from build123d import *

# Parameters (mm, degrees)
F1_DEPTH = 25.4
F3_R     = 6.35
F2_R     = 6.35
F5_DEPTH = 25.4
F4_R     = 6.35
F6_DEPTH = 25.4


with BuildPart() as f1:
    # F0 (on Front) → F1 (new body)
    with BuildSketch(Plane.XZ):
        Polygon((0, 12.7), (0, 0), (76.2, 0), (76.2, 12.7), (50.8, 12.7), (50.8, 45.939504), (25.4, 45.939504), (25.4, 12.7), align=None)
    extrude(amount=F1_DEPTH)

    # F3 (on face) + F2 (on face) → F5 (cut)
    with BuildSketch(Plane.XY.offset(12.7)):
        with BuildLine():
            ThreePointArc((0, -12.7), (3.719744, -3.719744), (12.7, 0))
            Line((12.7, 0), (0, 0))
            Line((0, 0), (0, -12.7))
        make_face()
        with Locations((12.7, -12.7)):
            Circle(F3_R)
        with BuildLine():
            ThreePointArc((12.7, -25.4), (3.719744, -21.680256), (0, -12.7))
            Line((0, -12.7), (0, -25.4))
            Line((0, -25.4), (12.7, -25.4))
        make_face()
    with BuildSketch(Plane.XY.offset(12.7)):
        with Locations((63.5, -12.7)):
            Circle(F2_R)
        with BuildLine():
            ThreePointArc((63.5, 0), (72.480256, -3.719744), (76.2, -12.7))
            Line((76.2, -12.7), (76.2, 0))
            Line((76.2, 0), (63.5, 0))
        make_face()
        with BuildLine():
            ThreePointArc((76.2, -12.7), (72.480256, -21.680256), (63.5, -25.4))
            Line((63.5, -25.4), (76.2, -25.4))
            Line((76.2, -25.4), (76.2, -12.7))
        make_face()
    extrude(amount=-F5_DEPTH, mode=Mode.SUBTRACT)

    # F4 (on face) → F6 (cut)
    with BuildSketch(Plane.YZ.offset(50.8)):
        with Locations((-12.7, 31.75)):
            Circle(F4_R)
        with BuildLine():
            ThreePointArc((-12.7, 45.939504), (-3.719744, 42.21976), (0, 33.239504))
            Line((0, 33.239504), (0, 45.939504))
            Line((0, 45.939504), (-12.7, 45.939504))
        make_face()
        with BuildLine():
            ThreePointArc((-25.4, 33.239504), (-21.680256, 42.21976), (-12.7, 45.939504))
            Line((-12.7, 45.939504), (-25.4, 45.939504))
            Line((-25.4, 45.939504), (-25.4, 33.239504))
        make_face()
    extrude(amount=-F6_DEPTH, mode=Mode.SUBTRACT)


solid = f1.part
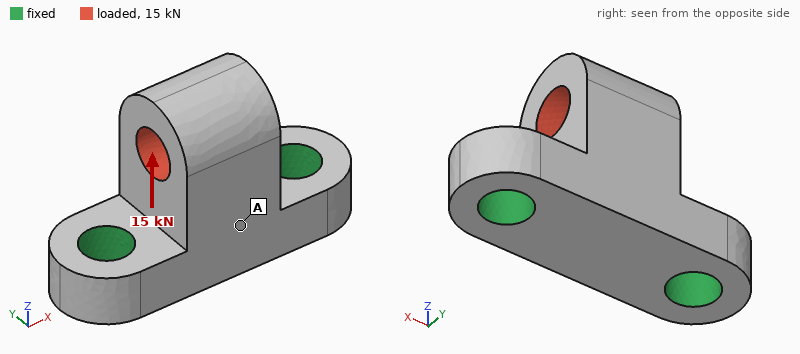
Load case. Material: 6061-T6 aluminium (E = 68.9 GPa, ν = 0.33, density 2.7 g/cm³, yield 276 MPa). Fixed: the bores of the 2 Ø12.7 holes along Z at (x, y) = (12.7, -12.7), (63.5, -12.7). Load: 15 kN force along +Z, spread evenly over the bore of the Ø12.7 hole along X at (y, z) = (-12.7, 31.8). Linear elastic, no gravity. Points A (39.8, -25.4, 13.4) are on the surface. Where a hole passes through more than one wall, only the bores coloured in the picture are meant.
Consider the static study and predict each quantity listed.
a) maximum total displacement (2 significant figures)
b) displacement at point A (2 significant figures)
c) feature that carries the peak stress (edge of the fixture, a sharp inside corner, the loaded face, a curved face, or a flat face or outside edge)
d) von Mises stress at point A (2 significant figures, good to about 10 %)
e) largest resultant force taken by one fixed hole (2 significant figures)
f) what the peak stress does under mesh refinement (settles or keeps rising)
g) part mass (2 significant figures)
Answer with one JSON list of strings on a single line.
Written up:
["33 µm", "21 µm", "edge of the fixture", "15 MPa", "7.8 kN", "keeps rising", "97 g"]
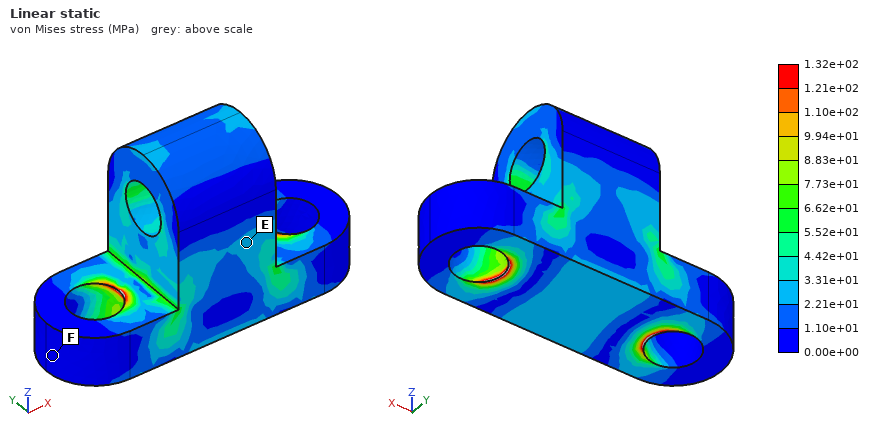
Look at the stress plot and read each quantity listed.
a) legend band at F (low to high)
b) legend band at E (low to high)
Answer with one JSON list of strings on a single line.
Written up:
["0.00e+00 to 1.10e+01 MPa", "2.21e+01 to 3.31e+01 MPa"]
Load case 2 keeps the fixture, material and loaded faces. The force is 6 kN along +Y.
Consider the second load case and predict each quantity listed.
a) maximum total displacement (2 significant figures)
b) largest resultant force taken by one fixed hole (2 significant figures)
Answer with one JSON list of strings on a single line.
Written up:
["0.14 mm", "3.0 kN"]
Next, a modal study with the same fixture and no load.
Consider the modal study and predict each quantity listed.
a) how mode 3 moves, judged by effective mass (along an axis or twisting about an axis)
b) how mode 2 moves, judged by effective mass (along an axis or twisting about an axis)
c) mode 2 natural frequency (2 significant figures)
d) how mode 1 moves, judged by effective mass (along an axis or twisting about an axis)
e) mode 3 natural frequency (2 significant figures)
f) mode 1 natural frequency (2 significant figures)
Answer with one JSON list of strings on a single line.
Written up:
["along Z", "along X", "11 kHz", "along Y", "17 kHz", "6500 Hz"]
